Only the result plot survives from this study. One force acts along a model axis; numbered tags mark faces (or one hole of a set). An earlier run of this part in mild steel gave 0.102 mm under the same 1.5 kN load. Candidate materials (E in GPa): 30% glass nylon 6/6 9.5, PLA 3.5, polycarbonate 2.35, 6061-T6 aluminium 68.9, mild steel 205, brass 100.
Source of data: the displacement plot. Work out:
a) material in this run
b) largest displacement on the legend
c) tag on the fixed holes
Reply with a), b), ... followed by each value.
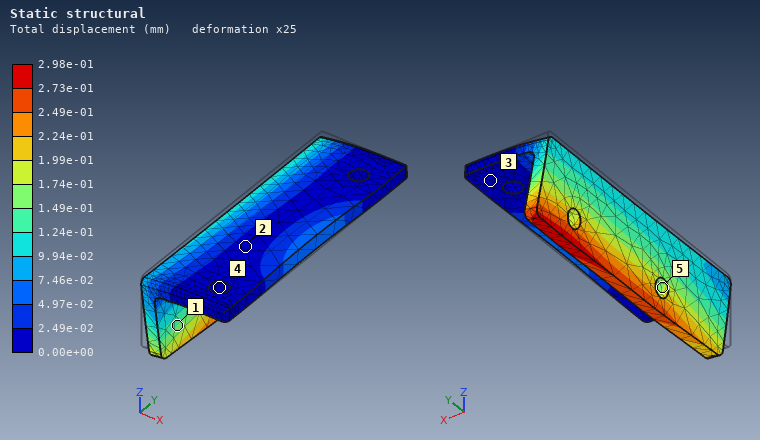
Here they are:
a) 6061-T6 aluminium
b) 2.98e-01 mm
c) 4
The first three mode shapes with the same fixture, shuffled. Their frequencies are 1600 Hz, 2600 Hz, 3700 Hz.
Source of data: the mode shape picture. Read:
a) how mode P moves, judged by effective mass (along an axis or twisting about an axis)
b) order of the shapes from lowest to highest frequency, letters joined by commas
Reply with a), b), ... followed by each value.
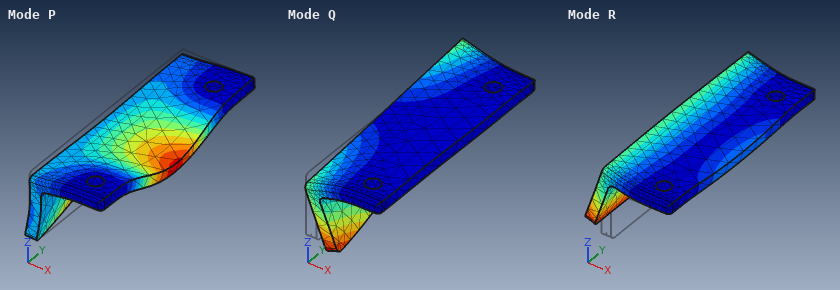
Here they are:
a) along Z
b) R, Q, P
